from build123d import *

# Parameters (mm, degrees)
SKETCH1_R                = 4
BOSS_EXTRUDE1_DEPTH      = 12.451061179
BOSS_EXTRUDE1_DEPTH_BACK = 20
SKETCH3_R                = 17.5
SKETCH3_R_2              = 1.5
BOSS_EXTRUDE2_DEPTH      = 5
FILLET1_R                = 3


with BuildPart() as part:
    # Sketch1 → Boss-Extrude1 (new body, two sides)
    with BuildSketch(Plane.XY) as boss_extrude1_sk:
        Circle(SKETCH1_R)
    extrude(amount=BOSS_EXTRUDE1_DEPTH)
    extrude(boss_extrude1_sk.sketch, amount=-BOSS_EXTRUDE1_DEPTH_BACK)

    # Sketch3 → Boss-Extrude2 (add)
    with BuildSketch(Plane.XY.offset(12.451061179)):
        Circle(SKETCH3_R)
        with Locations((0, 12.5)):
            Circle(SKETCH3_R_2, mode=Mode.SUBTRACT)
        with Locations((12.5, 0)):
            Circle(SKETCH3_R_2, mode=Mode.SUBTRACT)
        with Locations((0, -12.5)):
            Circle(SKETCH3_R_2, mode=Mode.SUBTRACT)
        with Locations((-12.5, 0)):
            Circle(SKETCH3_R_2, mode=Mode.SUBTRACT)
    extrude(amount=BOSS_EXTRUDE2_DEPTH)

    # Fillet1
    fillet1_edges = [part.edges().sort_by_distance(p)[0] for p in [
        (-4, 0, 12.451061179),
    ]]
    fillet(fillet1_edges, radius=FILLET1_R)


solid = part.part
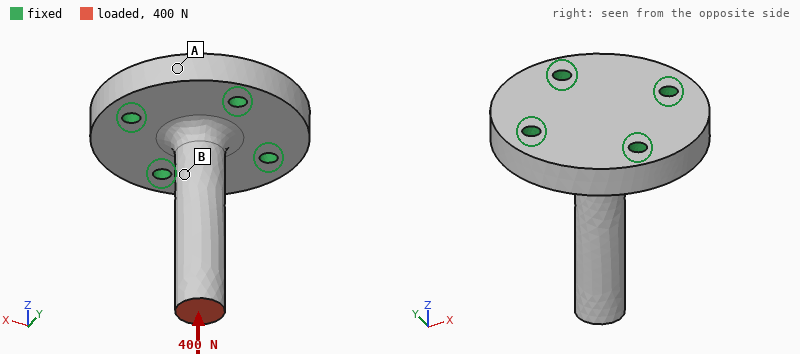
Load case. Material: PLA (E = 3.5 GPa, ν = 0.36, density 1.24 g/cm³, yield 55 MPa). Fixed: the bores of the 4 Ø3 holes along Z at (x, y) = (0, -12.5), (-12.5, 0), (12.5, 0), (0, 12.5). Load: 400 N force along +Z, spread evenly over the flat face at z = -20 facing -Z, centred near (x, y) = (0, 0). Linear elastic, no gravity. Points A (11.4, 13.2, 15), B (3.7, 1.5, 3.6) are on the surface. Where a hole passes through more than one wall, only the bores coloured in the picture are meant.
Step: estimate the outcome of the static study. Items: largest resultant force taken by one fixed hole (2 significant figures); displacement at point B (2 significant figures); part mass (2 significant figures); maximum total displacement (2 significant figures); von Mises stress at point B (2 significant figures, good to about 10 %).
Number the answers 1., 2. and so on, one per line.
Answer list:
1. 100 N
2. 46 µm
3. 7.9 g
4. 99 µm
5. 7.9 MPa
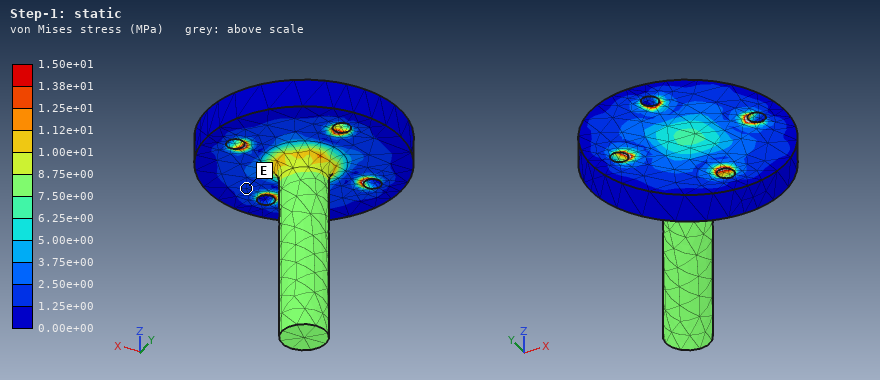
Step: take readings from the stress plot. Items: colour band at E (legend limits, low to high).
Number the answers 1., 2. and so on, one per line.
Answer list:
1. 1.25e+00 to 2.50e+00 MPa
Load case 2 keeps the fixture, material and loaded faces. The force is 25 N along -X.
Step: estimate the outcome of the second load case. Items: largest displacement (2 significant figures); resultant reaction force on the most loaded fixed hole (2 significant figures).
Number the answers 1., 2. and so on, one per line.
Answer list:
1. 0.45 mm
2. 39 N
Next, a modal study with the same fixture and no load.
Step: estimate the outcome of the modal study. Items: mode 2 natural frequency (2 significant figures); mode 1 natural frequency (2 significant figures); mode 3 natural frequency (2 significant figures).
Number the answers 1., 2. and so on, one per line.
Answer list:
1. 1700 Hz
2. 1700 Hz
3. 7900 Hz
